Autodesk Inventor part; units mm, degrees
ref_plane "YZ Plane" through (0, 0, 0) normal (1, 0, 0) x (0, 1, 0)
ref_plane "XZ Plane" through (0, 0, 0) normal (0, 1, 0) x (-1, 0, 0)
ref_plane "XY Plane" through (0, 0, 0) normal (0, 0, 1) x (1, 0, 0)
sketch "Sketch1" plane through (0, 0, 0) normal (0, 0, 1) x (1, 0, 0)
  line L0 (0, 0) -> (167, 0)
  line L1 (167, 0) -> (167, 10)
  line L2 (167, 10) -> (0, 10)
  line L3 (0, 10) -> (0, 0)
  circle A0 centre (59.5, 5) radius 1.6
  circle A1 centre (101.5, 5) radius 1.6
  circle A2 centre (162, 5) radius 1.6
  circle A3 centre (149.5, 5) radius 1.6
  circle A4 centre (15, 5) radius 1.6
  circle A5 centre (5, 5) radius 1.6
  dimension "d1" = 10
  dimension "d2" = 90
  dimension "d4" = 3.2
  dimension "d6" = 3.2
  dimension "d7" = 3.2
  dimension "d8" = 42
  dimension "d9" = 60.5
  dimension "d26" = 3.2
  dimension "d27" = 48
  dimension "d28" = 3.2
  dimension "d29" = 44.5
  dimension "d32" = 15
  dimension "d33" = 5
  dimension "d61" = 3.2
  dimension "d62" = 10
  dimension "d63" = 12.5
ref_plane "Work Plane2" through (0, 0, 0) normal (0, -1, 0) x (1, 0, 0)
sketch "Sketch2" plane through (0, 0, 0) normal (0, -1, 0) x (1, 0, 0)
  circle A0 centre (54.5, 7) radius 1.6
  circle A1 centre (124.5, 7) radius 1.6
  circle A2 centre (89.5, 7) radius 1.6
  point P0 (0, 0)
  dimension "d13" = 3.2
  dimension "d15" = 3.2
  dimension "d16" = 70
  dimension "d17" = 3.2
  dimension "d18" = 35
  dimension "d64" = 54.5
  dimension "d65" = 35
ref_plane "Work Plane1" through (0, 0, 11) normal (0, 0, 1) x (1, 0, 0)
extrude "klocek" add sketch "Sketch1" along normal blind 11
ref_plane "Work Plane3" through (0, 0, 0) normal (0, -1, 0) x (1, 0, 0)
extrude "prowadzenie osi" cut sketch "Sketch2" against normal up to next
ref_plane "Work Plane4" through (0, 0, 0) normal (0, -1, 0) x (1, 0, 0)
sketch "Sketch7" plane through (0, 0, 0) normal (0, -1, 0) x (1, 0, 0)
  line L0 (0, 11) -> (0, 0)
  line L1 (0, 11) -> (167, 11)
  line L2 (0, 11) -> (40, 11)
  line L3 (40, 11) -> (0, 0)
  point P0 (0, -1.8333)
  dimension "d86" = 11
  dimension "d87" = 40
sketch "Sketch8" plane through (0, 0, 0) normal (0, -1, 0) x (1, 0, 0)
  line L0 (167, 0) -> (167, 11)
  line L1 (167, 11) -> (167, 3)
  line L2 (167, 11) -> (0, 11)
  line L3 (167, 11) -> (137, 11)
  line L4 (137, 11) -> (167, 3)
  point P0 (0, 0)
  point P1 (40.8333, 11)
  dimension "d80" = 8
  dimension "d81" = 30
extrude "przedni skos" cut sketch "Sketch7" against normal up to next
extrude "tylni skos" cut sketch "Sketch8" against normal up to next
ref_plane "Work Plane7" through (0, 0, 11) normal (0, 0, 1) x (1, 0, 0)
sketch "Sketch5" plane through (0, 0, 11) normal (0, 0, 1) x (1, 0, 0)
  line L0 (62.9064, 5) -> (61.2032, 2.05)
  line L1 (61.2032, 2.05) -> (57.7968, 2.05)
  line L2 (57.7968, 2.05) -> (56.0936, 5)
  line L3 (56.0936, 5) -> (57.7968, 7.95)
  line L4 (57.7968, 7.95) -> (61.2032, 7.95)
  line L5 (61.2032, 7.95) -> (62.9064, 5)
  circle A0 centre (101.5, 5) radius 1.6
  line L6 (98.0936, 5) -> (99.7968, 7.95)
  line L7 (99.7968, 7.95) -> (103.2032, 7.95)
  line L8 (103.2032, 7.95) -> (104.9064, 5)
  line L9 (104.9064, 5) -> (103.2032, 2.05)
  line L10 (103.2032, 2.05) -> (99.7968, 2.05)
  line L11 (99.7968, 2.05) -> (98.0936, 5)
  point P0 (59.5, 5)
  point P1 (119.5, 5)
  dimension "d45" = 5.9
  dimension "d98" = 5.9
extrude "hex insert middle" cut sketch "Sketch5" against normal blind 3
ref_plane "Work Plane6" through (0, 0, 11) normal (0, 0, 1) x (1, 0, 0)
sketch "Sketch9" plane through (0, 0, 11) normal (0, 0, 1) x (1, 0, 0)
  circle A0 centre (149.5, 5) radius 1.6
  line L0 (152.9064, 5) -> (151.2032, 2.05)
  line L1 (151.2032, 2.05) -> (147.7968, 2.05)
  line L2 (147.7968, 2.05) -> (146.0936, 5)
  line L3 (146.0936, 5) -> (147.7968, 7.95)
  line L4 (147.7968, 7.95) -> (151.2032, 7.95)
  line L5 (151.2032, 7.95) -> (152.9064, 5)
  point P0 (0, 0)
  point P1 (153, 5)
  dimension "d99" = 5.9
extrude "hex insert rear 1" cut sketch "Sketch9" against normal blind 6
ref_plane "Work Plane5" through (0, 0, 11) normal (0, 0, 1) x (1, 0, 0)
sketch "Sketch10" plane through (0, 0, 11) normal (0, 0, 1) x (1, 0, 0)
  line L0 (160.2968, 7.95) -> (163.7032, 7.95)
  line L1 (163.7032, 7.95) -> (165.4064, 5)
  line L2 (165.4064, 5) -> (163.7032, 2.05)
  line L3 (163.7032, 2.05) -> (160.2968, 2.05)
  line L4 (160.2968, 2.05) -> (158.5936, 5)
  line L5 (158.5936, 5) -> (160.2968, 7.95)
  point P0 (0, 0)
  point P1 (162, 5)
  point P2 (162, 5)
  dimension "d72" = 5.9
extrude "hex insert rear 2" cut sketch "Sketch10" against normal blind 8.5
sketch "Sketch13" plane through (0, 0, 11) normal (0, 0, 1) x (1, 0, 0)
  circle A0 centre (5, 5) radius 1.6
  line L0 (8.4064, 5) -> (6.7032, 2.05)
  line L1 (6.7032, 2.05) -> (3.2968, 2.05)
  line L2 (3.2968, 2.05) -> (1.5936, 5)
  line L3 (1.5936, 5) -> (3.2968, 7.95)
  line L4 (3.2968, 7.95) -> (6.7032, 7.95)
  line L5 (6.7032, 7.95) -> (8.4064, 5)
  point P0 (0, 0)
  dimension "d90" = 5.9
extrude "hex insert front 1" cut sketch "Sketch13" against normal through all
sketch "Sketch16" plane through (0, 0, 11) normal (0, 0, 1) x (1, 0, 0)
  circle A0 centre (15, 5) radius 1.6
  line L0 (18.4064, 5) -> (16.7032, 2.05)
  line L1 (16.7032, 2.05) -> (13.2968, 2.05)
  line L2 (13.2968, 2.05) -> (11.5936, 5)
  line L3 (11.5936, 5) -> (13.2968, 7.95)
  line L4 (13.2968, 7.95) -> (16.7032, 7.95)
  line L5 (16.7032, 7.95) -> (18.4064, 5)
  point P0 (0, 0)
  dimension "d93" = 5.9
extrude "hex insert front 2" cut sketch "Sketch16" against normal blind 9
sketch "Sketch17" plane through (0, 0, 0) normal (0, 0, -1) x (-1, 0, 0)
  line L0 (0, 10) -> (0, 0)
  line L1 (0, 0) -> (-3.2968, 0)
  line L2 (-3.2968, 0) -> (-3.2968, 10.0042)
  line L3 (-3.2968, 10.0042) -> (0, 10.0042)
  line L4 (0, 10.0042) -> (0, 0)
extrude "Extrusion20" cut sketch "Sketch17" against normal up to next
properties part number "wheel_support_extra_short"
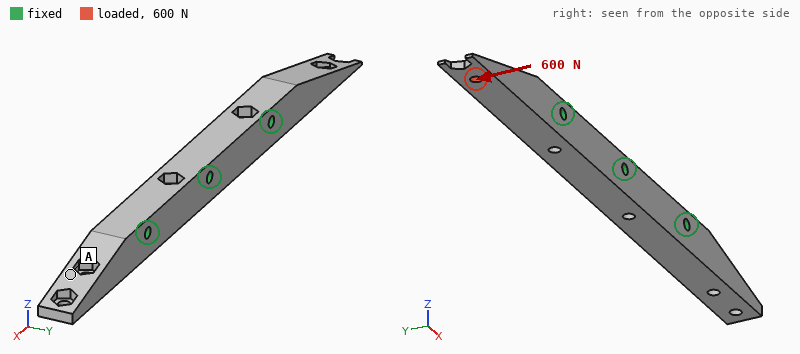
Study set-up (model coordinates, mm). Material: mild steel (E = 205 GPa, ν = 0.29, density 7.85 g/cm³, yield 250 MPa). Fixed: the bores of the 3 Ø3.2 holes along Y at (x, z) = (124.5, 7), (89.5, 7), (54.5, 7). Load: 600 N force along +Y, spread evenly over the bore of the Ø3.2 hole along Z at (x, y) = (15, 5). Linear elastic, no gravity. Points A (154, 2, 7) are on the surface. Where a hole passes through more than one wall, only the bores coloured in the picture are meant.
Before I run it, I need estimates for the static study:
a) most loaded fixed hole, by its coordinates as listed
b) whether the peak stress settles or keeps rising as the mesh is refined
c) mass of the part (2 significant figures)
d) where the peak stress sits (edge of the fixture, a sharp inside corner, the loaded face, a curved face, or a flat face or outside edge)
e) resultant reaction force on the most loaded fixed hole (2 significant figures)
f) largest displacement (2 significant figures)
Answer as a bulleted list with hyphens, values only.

- (54.5, 7)
- keeps rising
- 110 g
- edge of the fixture
- 700 N
- 0.12 mm
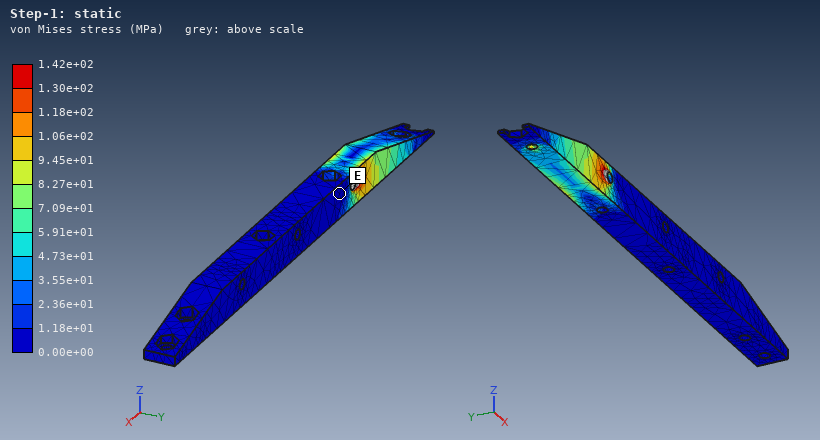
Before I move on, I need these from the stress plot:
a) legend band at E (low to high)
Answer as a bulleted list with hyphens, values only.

- 0.00e+00 to 1.18e+01 MPa
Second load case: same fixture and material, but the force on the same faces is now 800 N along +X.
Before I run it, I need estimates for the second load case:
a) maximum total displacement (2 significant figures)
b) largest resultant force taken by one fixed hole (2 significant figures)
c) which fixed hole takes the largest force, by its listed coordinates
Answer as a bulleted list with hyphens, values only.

- 35 µm
- 640 N
- (54.5, 7)
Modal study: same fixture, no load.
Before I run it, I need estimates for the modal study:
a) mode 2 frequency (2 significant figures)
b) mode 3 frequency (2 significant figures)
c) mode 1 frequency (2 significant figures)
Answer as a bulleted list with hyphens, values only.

- 5400 Hz
- 5900 Hz
- 5000 Hz
